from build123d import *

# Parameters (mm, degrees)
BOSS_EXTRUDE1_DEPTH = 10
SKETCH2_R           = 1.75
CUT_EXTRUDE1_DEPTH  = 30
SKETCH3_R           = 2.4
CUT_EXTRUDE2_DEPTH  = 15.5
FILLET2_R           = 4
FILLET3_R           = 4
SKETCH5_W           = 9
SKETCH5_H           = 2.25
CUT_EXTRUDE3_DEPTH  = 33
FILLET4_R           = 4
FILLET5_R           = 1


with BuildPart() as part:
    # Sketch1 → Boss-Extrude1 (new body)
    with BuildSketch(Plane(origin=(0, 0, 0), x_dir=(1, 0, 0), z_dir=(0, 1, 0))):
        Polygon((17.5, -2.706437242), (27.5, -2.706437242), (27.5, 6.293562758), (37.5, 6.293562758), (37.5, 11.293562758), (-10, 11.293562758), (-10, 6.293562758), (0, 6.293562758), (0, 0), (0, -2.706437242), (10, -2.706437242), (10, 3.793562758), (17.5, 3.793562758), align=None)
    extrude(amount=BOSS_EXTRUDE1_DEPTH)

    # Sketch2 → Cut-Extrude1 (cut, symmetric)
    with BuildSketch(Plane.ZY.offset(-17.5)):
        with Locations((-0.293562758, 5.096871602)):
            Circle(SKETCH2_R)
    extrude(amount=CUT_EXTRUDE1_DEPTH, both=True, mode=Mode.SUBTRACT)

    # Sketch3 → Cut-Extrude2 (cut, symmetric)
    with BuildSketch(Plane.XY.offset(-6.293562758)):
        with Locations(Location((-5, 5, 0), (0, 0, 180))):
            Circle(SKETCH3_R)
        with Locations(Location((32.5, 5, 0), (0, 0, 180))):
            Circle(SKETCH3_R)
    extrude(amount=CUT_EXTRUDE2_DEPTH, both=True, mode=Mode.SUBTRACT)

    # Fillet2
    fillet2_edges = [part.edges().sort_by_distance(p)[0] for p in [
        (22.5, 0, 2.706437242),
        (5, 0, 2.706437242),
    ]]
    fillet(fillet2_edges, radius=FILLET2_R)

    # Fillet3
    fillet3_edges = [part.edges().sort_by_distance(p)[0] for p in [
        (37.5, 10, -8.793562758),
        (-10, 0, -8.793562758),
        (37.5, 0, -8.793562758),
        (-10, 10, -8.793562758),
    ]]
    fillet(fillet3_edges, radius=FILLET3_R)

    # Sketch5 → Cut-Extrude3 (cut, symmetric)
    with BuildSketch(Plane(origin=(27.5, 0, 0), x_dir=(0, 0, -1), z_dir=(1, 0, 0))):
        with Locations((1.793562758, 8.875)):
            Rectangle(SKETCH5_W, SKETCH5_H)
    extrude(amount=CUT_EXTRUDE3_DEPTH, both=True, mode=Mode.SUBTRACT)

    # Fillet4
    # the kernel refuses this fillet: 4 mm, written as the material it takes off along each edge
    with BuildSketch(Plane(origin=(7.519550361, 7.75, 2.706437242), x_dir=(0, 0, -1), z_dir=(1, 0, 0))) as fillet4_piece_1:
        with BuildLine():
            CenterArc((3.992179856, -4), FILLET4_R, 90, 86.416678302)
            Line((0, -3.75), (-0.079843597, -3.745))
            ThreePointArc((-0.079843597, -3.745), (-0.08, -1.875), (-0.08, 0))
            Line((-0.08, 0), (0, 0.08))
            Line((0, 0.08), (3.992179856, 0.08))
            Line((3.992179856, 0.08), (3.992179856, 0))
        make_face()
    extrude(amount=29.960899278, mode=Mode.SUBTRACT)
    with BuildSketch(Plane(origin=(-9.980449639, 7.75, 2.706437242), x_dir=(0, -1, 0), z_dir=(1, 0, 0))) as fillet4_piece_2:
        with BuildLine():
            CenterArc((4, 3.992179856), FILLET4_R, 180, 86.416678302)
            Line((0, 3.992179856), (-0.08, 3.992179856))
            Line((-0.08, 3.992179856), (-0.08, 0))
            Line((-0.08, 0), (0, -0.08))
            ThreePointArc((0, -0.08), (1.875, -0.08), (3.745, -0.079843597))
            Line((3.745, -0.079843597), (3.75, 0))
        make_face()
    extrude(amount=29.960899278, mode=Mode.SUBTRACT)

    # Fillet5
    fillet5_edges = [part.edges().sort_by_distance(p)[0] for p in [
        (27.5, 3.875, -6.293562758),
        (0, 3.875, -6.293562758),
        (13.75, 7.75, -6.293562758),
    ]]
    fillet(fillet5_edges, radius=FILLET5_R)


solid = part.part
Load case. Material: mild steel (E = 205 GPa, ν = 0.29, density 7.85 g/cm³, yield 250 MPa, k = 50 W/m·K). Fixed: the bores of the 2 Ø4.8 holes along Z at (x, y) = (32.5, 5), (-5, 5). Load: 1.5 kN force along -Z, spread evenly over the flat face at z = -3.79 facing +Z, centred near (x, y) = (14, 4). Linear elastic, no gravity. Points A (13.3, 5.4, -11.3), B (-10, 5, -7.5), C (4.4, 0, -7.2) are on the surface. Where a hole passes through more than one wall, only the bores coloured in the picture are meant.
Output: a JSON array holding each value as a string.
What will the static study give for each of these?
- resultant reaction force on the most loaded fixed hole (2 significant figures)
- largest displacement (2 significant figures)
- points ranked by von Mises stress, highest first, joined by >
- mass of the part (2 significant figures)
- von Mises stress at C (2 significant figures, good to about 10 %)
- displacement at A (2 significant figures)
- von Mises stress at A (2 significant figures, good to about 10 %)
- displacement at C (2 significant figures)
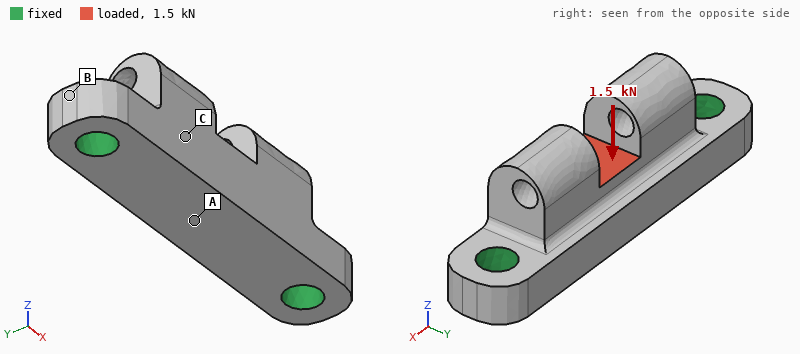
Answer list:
["920 N", "11 µm", "A > C > B", "26 g", "34 MPa", "9.2 µm", "69 MPa", "5.7 µm"]
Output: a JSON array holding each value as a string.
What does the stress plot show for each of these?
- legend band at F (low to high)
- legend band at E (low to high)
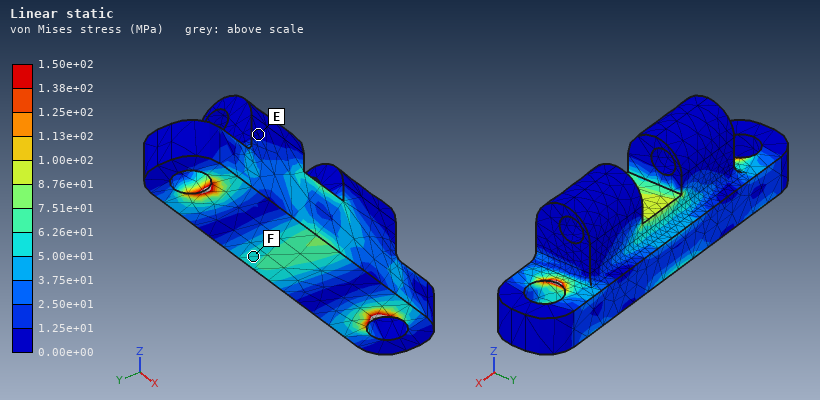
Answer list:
["5.00e+01 to 6.26e+01 MPa", "0.00e+00 to 1.25e+01 MPa"]
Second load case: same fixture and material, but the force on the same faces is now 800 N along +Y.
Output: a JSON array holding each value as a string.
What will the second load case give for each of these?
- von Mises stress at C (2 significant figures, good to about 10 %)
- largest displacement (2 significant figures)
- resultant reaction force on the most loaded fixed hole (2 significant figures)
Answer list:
["14 MPa", "8.1 µm", "400 N"]
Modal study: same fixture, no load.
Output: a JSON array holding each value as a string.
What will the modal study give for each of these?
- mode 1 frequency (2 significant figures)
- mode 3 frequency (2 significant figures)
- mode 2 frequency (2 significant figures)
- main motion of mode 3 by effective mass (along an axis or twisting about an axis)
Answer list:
["17 kHz", "28 kHz", "19 kHz", "along Y"]
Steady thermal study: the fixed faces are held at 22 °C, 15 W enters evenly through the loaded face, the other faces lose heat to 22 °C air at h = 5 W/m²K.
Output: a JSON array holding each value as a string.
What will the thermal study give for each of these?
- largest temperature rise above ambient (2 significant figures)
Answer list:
["46 K"]
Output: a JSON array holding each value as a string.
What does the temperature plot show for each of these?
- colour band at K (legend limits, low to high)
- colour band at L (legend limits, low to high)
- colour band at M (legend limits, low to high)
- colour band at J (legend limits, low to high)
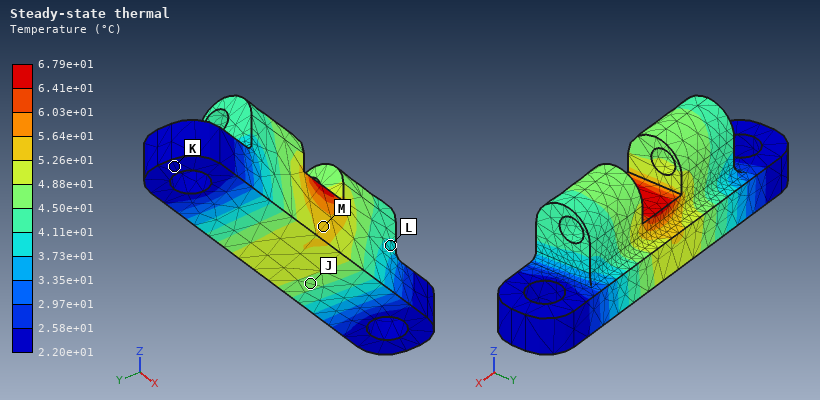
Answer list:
["2.20e+01 to 2.58e+01 °C", "3.73e+01 to 4.11e+01 °C", "5.26e+01 to 5.64e+01 °C", "4.50e+01 to 4.88e+01 °C"]
